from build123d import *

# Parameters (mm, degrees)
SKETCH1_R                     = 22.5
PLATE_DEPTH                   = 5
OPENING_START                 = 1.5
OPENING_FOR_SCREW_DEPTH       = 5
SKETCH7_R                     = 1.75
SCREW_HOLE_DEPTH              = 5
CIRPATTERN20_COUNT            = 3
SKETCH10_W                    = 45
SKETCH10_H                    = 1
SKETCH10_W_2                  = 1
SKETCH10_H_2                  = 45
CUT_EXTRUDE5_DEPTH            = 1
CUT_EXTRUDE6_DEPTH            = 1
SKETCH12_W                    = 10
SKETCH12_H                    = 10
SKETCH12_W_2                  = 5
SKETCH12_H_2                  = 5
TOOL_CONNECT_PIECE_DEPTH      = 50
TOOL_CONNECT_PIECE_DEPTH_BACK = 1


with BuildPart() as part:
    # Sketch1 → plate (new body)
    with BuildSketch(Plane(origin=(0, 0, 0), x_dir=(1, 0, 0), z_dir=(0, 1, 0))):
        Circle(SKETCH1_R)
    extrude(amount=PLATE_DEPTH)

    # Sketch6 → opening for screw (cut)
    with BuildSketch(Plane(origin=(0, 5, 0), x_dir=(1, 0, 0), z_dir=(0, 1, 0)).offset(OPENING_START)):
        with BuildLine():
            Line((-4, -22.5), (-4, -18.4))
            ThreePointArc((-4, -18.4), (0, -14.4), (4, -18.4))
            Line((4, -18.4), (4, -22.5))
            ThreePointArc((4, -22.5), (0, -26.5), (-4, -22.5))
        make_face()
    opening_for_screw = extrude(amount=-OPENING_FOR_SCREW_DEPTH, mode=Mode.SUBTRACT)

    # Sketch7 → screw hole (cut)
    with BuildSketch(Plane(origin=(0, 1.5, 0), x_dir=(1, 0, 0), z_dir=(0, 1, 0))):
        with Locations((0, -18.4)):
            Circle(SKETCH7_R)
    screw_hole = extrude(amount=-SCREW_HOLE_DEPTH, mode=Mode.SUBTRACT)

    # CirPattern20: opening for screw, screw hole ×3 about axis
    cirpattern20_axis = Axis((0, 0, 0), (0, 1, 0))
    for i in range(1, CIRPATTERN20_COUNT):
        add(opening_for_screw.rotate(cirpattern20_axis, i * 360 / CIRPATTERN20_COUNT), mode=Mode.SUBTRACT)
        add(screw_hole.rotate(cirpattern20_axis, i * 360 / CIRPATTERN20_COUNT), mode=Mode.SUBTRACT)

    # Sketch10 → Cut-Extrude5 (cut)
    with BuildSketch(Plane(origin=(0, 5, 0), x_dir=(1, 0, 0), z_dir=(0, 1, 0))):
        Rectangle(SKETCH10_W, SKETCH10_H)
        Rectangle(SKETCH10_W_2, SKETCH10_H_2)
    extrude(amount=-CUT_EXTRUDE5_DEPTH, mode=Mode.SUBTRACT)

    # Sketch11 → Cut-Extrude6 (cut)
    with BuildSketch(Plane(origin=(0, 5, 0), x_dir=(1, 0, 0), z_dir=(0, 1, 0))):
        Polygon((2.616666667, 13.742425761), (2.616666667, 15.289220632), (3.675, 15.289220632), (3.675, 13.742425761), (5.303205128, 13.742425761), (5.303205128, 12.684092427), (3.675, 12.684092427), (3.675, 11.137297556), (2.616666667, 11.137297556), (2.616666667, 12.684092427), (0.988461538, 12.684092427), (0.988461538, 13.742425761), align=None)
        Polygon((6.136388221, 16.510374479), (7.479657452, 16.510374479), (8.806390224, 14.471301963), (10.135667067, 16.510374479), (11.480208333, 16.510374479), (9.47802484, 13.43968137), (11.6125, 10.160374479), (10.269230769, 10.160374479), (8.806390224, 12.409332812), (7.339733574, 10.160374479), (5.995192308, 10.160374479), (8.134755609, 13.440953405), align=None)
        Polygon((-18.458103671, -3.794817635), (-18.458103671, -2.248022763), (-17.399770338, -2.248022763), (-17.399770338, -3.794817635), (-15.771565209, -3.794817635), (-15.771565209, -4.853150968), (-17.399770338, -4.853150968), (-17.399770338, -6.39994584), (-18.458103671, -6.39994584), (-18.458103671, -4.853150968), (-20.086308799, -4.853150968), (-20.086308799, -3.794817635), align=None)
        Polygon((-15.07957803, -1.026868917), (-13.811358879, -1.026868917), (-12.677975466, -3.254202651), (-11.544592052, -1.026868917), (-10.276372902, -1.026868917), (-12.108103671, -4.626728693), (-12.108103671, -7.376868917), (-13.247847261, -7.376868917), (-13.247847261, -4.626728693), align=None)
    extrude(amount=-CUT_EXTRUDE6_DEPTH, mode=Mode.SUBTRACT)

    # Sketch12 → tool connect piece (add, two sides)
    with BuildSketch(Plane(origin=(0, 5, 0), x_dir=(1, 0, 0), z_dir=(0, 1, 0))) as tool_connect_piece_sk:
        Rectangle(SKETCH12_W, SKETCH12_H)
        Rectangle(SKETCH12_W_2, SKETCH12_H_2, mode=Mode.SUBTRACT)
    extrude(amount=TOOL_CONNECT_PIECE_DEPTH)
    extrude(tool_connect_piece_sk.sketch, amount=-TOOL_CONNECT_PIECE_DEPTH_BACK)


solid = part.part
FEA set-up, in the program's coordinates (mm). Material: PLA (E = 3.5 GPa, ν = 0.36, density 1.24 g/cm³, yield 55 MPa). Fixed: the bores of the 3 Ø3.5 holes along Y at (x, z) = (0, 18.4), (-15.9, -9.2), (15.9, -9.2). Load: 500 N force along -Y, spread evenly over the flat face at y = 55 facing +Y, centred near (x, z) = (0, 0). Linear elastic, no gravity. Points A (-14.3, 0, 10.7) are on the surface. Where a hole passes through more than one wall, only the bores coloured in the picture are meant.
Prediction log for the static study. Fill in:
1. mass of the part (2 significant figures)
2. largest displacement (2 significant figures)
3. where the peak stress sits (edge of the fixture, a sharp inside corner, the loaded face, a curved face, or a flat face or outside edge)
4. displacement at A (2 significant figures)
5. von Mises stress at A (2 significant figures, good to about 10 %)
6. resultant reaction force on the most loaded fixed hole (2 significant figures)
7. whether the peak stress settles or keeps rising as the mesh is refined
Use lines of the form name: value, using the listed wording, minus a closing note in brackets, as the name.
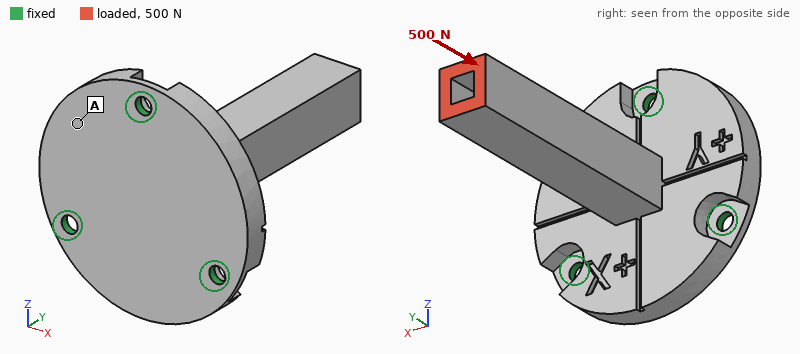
mass of the part: 14 g
largest displacement: 0.26 mm
where the peak stress sits: edge of the fixture
displacement at A: 0.082 mm
von Mises stress at A: 5.9 MPa
resultant reaction force on the most loaded fixed hole: 240 N
whether the peak stress settles or keeps rising as the mesh is refined: keeps rising
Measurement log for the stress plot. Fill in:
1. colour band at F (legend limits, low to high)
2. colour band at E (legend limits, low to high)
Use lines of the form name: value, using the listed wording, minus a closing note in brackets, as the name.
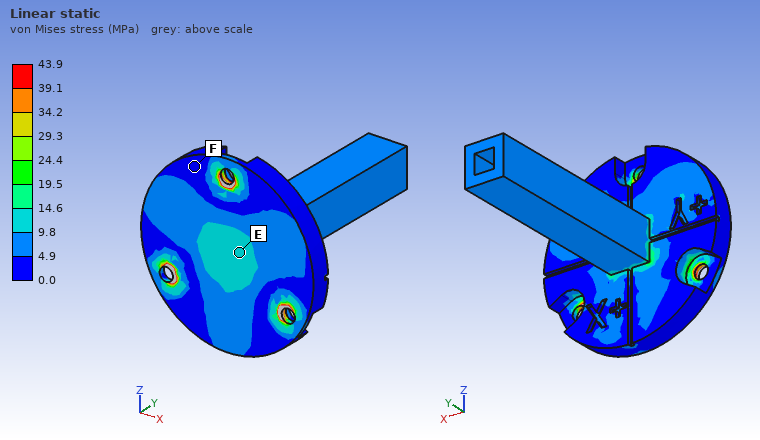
colour band at F: 0.0 to 4.9 MPa
colour band at E: 9.8 to 14.6 MPa
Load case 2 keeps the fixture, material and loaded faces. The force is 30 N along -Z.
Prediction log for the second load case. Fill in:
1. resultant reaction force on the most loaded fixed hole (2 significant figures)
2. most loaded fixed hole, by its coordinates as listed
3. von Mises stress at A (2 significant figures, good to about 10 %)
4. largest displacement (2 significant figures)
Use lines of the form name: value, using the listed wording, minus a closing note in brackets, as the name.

resultant reaction force on the most loaded fixed hole: 78 N
most loaded fixed hole, by its coordinates as listed: (0, 18.4)
von Mises stress at A: 1.4 MPa
largest displacement: 0.76 mm
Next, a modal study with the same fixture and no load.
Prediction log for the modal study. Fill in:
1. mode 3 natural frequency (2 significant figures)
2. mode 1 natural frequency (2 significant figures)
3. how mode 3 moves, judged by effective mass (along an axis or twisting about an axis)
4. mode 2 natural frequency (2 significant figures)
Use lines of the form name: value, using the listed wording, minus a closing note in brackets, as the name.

mode 3 natural frequency: 3000 Hz
mode 1 natural frequency: 860 Hz
how mode 3 moves, judged by effective mass: along Y
mode 2 natural frequency: 860 Hz
